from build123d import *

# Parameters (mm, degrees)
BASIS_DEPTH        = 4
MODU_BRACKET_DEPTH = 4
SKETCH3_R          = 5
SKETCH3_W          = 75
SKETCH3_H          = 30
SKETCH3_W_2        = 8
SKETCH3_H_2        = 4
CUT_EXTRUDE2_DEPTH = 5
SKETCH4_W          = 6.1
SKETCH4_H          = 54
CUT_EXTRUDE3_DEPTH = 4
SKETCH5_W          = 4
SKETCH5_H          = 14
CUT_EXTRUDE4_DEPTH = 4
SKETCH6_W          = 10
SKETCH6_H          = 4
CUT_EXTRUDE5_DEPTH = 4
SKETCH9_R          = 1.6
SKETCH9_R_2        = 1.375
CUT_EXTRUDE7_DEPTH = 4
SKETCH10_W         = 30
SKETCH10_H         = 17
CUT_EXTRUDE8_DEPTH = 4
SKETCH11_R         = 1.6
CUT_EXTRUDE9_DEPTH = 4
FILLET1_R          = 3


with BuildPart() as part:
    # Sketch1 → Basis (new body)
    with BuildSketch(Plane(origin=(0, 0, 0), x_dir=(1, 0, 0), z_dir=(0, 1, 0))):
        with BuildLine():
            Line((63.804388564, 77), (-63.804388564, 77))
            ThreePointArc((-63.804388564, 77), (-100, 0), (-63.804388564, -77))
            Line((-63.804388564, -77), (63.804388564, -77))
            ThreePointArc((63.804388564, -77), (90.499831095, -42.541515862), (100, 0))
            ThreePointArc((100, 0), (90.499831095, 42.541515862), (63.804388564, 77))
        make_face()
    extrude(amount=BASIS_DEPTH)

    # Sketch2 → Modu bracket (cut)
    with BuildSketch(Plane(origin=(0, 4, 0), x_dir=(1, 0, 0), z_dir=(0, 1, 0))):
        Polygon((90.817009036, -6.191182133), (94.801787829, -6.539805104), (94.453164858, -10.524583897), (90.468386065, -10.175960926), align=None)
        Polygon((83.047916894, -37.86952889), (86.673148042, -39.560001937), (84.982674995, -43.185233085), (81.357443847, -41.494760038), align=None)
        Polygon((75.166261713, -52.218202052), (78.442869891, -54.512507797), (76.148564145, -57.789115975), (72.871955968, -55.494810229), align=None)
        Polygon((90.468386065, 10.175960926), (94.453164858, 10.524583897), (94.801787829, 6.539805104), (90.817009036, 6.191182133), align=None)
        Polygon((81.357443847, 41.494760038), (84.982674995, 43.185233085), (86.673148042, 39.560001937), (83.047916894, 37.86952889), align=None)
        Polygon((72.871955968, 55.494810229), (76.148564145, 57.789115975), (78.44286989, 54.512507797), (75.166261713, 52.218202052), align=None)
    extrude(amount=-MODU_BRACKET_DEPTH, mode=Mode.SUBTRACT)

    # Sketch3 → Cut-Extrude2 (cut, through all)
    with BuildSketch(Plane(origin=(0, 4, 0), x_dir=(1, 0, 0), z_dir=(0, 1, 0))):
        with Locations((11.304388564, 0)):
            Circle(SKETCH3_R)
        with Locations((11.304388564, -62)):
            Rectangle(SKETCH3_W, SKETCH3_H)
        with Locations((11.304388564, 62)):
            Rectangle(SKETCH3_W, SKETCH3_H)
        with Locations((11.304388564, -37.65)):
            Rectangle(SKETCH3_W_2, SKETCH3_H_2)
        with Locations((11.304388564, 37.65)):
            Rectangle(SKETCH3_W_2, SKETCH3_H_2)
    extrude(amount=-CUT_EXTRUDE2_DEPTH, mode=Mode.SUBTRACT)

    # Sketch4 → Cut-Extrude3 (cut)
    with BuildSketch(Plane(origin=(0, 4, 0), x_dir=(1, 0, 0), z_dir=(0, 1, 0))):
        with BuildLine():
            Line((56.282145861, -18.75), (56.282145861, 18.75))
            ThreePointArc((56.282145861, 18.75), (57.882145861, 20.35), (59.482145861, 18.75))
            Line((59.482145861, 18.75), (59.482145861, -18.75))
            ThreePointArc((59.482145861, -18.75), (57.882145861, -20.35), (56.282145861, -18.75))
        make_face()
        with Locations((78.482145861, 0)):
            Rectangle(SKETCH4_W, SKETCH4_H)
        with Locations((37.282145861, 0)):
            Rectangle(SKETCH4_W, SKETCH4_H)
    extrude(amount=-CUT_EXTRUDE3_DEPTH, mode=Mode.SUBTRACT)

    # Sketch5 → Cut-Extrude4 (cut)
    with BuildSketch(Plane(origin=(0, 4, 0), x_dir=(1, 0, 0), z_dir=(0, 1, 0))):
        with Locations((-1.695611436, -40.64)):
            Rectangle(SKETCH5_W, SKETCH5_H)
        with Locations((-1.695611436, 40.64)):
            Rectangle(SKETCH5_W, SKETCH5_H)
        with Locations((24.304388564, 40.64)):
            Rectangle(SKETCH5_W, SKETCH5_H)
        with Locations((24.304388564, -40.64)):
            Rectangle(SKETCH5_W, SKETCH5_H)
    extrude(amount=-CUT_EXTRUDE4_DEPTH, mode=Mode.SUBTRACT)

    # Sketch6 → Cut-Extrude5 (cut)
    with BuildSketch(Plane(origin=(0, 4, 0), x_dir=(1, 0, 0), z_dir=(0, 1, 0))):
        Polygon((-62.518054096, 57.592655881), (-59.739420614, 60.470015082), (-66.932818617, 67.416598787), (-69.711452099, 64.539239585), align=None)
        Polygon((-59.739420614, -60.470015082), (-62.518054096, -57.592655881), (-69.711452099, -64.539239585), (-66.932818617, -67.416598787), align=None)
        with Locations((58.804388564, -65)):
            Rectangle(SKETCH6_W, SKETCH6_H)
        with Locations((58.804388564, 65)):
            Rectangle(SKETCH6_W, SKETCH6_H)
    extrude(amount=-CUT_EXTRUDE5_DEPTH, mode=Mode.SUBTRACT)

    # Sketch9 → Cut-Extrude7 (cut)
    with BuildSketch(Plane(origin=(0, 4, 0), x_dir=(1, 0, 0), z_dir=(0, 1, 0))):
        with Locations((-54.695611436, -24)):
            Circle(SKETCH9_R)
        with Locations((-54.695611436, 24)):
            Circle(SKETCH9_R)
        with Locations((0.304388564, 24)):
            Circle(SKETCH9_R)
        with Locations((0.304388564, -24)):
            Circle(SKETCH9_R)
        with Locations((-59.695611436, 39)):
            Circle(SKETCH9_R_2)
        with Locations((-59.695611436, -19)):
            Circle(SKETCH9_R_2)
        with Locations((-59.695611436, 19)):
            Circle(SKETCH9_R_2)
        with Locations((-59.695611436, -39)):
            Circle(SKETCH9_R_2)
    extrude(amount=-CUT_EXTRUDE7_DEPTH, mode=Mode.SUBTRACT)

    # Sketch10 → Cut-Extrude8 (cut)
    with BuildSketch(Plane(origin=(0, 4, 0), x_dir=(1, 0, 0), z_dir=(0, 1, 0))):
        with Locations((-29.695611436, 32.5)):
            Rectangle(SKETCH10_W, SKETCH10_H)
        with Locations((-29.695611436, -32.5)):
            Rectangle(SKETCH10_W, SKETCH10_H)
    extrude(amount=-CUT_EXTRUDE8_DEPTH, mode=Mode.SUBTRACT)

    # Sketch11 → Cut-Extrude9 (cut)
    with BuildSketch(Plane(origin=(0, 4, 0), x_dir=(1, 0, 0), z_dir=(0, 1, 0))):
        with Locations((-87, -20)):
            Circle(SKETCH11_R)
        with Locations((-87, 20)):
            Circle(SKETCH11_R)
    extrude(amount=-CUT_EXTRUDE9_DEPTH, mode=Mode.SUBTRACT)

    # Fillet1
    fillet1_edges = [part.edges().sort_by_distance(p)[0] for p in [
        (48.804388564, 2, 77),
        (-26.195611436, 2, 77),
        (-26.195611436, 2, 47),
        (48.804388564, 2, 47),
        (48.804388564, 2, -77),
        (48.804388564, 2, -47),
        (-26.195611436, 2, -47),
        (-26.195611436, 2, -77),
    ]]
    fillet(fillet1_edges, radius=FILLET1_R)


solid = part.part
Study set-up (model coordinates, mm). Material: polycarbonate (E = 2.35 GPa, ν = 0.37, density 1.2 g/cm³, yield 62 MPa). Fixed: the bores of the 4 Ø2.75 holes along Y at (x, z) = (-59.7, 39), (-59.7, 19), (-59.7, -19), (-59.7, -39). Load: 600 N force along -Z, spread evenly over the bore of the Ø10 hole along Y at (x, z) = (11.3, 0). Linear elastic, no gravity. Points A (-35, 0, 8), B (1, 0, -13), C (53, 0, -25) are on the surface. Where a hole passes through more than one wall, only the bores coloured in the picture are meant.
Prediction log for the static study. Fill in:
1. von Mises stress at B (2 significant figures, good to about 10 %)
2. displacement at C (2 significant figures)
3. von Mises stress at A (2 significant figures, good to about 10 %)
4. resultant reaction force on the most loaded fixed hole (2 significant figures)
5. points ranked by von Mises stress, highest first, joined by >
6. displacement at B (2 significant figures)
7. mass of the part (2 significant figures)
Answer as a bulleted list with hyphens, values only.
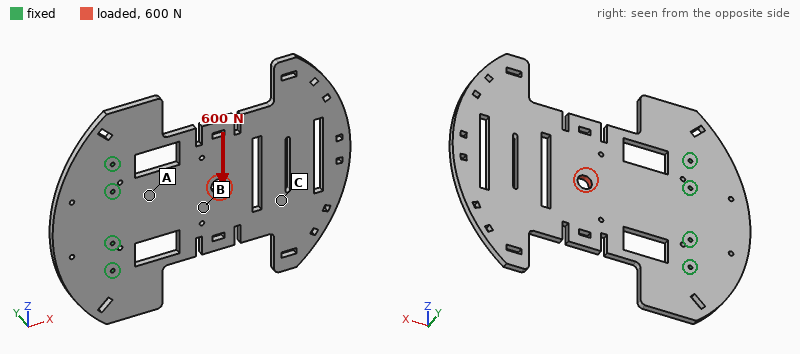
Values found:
- 3.7 MPa
- 0.71 mm
- 5.4 MPa
- 430 N
- A > B > C
- 0.38 mm
- 98 g
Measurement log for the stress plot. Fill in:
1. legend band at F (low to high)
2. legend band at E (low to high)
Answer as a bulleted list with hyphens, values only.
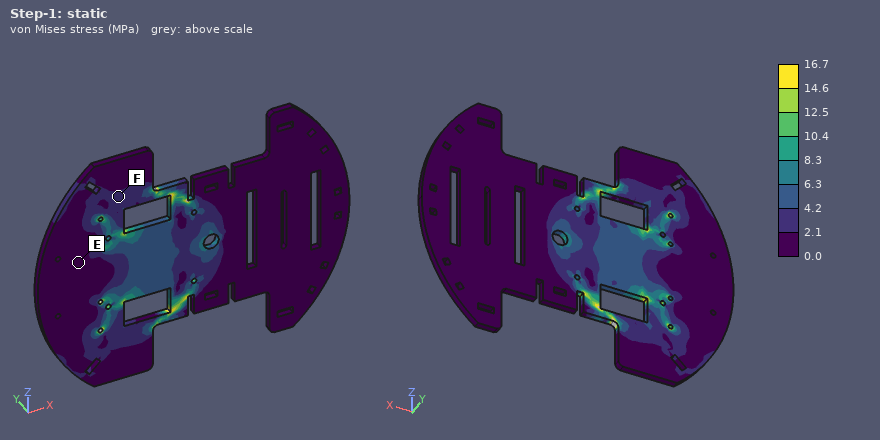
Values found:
- 2.1 to 4.2 MPa
- 0.0 to 2.1 MPa
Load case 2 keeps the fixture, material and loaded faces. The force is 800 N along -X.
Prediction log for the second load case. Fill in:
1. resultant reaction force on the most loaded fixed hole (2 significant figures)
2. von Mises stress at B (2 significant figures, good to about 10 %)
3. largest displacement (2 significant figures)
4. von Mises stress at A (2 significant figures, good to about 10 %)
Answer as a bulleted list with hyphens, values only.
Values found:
- 280 N
- 3.6 MPa
- 0.16 mm
- 3.2 MPa
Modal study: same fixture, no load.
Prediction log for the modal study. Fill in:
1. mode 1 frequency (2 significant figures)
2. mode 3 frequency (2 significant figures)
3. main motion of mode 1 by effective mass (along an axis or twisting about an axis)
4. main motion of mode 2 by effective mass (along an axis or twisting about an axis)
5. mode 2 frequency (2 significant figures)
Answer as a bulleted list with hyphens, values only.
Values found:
- 31 Hz
- 180 Hz
- along Y
- twisting about X
- 84 Hz
